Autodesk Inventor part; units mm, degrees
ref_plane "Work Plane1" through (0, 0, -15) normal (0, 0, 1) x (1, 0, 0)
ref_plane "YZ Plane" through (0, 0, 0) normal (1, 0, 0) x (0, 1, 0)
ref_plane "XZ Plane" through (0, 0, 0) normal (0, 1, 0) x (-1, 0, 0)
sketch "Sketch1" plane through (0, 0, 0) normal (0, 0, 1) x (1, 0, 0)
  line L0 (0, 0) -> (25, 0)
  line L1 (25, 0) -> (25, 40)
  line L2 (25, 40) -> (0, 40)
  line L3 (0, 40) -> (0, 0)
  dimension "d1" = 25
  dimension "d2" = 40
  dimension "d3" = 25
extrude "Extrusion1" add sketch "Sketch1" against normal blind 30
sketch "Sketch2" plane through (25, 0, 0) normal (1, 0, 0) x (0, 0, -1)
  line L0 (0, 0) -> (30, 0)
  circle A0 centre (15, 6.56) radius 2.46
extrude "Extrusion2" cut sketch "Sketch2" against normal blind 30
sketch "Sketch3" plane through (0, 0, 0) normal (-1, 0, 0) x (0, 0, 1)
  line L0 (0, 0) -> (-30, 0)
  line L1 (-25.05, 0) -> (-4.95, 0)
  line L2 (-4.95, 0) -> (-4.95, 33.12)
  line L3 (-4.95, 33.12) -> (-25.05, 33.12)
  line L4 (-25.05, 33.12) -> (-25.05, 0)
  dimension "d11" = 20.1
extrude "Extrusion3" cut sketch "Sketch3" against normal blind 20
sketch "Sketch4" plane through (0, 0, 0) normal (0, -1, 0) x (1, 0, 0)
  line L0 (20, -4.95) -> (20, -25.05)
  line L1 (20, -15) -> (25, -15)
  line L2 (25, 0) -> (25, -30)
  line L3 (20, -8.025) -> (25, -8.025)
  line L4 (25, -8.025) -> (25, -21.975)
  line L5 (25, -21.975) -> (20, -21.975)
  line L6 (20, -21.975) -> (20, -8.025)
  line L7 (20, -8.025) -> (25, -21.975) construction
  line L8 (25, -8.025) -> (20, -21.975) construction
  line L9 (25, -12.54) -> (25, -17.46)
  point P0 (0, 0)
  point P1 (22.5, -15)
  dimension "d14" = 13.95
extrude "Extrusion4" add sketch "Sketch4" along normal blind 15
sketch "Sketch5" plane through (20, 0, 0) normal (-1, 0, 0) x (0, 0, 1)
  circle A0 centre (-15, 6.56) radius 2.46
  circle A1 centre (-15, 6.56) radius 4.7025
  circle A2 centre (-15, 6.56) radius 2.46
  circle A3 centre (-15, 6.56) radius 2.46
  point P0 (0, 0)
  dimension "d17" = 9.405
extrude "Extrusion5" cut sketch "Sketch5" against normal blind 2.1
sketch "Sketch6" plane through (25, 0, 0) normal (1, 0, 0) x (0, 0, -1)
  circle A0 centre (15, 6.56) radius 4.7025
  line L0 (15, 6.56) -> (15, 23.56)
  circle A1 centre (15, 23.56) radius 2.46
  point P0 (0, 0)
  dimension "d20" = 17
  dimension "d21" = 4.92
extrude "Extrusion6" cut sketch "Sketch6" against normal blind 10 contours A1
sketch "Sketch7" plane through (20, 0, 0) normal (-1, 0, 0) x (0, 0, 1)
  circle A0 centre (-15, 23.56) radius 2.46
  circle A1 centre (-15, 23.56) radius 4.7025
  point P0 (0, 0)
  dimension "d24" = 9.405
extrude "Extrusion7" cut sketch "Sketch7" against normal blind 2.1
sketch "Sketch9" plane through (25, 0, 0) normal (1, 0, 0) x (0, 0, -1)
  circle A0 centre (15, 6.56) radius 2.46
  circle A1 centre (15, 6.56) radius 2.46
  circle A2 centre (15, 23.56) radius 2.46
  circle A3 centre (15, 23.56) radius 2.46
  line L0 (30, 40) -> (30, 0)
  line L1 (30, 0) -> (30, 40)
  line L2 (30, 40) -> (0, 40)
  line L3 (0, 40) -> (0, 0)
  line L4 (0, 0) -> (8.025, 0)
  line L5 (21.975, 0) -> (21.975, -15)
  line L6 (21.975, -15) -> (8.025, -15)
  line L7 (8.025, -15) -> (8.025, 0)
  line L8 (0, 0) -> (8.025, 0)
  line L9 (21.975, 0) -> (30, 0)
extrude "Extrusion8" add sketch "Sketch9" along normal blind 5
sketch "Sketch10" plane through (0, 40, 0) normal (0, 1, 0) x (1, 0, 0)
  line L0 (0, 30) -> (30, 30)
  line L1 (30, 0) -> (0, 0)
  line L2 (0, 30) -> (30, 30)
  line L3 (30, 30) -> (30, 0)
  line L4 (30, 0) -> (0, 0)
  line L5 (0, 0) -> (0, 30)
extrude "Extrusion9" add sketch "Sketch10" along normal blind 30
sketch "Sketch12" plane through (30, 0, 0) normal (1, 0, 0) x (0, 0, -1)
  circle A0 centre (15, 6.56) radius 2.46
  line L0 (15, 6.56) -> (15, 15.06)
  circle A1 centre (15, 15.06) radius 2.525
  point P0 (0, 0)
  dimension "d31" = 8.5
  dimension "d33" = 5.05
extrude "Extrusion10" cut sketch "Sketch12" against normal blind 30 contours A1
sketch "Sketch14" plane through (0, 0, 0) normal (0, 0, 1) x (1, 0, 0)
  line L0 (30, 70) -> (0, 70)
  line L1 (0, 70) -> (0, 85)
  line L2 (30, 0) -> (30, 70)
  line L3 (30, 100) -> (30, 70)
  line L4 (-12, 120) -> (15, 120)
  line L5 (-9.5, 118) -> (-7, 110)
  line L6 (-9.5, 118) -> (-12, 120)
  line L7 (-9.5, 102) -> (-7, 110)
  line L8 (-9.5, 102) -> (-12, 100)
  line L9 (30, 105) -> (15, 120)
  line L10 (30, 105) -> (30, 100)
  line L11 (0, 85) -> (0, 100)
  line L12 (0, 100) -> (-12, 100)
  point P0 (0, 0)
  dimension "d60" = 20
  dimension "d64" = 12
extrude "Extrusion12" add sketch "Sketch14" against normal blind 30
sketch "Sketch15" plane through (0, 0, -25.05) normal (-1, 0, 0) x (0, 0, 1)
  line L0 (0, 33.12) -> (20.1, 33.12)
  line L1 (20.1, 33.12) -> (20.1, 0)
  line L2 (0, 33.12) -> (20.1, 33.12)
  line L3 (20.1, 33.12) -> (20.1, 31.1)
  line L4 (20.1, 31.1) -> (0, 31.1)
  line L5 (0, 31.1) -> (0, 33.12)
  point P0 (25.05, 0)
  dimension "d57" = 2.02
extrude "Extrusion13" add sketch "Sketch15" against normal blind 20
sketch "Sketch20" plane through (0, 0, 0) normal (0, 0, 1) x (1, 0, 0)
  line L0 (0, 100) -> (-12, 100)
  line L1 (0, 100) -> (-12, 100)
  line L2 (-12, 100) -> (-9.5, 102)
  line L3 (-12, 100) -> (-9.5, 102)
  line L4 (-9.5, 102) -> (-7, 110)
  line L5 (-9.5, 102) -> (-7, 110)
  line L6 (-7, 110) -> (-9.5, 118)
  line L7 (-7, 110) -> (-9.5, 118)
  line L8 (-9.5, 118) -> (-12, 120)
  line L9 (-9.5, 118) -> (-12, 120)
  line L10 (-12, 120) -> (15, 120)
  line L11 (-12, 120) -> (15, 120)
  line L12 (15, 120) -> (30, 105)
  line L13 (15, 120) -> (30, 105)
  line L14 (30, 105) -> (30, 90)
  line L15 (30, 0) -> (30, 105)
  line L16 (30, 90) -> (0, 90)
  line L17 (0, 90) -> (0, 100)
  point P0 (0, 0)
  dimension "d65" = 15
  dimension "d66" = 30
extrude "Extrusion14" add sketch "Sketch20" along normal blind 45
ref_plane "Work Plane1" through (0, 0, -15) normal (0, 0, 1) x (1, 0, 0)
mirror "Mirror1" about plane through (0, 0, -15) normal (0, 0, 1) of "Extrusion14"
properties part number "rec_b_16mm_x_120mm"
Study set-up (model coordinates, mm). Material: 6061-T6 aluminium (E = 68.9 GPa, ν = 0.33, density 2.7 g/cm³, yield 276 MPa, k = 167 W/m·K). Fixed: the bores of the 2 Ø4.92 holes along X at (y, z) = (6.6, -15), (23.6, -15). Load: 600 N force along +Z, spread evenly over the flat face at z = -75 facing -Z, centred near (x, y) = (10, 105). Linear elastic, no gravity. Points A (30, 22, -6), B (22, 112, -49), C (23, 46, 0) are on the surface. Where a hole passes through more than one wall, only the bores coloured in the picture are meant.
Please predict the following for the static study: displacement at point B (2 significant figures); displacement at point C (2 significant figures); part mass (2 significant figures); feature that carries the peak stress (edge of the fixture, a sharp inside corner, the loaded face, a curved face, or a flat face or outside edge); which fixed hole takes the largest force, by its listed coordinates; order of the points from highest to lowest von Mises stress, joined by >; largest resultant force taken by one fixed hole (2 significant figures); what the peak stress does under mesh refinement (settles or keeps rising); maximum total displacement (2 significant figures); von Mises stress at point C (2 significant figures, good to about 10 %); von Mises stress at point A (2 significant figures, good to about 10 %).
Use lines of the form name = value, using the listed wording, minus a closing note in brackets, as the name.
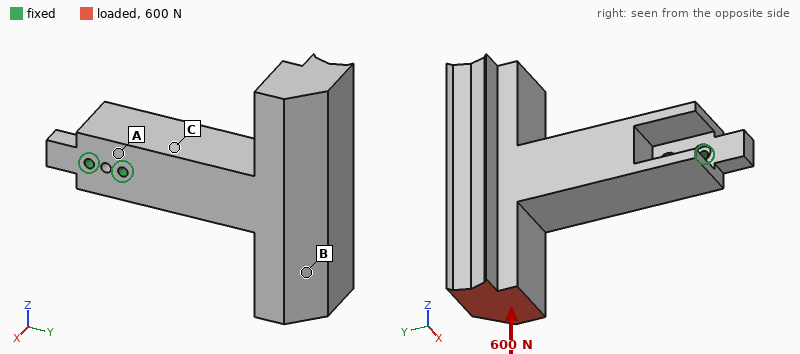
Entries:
displacement at point B = 0.094 mm
displacement at point C = 0.022 mm
part mass = 500 g
feature that carries the peak stress = edge of the fixture
which fixed hole takes the largest force, by its listed coordinates = (23.6, -15)
order of the points from highest to lowest von Mises stress, joined by > = A > C > B
largest resultant force taken by one fixed hole = 2.7 kN
what the peak stress does under mesh refinement = keeps rising
maximum total displacement = 0.12 mm
von Mises stress at point C = 9.3 MPa
von Mises stress at point A = 16 MPa
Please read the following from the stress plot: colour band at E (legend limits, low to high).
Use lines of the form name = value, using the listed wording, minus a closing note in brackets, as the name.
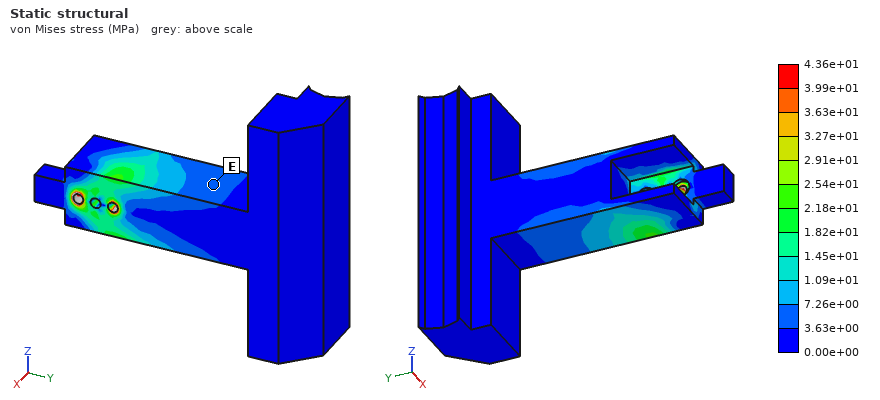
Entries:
colour band at E = 3.63e+00 to 7.26e+00 MPa
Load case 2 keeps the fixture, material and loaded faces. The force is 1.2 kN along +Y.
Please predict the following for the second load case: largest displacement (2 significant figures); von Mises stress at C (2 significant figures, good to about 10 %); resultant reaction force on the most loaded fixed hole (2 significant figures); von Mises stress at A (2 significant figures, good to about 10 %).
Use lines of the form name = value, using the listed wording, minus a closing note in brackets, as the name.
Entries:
largest displacement = 0.24 mm
von Mises stress at C = 20 MPa
resultant reaction force on the most loaded fixed hole = 3.3 kN
von Mises stress at A = 27 MPa
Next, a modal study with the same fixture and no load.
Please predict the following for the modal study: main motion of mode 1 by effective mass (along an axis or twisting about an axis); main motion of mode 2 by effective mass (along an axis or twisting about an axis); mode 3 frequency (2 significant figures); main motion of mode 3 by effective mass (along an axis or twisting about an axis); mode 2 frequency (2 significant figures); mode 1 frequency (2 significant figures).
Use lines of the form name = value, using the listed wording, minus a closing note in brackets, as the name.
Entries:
main motion of mode 1 by effective mass = along X
main motion of mode 2 by effective mass = along Z
mode 3 frequency = 930 Hz
main motion of mode 3 by effective mass = twisting about Y
mode 2 frequency = 670 Hz
mode 1 frequency = 620 Hz
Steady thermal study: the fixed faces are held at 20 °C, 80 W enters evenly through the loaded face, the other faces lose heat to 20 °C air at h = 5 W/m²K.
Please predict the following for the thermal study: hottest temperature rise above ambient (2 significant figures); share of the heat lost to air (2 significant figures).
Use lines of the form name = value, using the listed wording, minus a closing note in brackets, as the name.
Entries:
hottest temperature rise above ambient = 77 K
share of the heat lost to air = 7.5 %
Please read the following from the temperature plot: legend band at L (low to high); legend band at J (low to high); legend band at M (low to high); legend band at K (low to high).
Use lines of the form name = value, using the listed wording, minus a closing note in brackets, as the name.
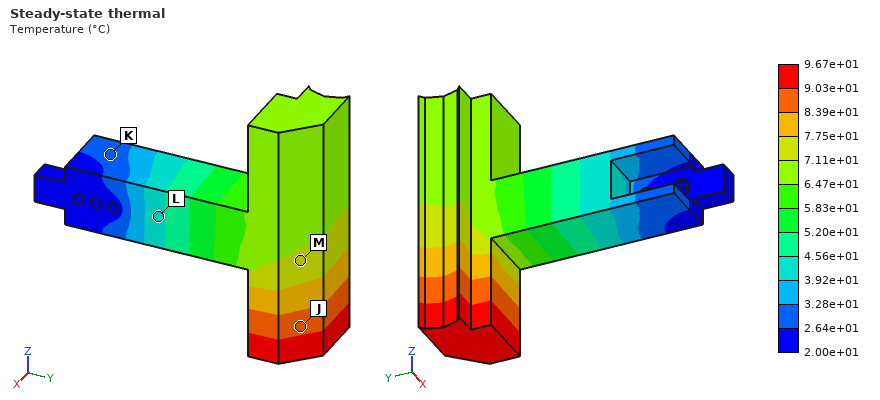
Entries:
legend band at L = 3.92e+01 to 4.56e+01 °C
legend band at J = 8.39e+01 to 9.03e+01 °C
legend band at M = 7.11e+01 to 7.75e+01 °C
legend band at K = 2.64e+01 to 3.28e+01 °C
